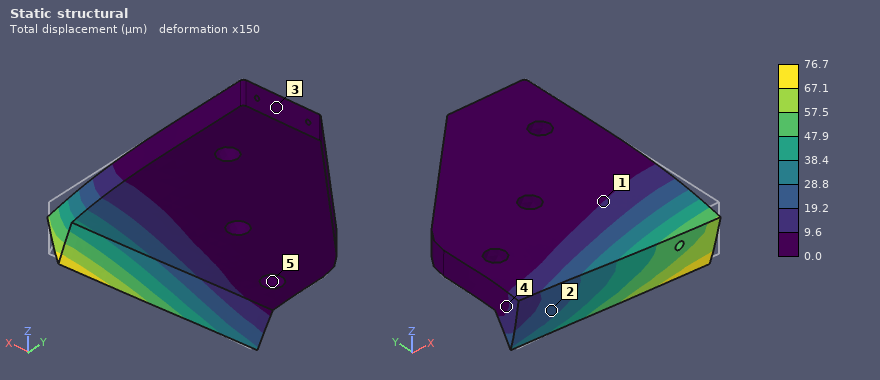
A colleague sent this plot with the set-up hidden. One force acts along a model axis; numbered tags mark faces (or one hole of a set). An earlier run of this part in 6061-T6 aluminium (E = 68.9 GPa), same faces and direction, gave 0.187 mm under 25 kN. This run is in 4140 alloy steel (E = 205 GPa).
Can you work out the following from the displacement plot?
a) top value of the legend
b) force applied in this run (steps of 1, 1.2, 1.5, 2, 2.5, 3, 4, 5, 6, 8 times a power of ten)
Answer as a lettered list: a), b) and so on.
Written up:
a) 76.7 µm
b) 30 kN
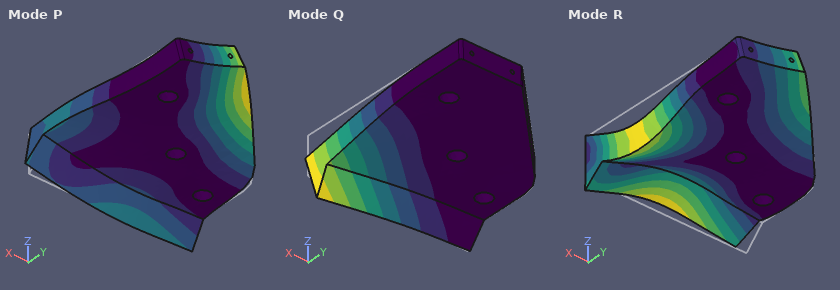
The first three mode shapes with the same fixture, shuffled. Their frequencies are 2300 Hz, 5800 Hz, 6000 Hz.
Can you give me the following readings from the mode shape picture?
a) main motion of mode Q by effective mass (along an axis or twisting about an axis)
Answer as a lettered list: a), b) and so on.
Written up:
a) along Z
